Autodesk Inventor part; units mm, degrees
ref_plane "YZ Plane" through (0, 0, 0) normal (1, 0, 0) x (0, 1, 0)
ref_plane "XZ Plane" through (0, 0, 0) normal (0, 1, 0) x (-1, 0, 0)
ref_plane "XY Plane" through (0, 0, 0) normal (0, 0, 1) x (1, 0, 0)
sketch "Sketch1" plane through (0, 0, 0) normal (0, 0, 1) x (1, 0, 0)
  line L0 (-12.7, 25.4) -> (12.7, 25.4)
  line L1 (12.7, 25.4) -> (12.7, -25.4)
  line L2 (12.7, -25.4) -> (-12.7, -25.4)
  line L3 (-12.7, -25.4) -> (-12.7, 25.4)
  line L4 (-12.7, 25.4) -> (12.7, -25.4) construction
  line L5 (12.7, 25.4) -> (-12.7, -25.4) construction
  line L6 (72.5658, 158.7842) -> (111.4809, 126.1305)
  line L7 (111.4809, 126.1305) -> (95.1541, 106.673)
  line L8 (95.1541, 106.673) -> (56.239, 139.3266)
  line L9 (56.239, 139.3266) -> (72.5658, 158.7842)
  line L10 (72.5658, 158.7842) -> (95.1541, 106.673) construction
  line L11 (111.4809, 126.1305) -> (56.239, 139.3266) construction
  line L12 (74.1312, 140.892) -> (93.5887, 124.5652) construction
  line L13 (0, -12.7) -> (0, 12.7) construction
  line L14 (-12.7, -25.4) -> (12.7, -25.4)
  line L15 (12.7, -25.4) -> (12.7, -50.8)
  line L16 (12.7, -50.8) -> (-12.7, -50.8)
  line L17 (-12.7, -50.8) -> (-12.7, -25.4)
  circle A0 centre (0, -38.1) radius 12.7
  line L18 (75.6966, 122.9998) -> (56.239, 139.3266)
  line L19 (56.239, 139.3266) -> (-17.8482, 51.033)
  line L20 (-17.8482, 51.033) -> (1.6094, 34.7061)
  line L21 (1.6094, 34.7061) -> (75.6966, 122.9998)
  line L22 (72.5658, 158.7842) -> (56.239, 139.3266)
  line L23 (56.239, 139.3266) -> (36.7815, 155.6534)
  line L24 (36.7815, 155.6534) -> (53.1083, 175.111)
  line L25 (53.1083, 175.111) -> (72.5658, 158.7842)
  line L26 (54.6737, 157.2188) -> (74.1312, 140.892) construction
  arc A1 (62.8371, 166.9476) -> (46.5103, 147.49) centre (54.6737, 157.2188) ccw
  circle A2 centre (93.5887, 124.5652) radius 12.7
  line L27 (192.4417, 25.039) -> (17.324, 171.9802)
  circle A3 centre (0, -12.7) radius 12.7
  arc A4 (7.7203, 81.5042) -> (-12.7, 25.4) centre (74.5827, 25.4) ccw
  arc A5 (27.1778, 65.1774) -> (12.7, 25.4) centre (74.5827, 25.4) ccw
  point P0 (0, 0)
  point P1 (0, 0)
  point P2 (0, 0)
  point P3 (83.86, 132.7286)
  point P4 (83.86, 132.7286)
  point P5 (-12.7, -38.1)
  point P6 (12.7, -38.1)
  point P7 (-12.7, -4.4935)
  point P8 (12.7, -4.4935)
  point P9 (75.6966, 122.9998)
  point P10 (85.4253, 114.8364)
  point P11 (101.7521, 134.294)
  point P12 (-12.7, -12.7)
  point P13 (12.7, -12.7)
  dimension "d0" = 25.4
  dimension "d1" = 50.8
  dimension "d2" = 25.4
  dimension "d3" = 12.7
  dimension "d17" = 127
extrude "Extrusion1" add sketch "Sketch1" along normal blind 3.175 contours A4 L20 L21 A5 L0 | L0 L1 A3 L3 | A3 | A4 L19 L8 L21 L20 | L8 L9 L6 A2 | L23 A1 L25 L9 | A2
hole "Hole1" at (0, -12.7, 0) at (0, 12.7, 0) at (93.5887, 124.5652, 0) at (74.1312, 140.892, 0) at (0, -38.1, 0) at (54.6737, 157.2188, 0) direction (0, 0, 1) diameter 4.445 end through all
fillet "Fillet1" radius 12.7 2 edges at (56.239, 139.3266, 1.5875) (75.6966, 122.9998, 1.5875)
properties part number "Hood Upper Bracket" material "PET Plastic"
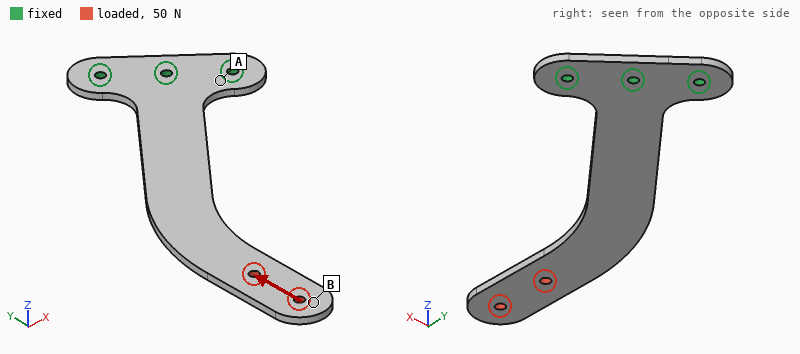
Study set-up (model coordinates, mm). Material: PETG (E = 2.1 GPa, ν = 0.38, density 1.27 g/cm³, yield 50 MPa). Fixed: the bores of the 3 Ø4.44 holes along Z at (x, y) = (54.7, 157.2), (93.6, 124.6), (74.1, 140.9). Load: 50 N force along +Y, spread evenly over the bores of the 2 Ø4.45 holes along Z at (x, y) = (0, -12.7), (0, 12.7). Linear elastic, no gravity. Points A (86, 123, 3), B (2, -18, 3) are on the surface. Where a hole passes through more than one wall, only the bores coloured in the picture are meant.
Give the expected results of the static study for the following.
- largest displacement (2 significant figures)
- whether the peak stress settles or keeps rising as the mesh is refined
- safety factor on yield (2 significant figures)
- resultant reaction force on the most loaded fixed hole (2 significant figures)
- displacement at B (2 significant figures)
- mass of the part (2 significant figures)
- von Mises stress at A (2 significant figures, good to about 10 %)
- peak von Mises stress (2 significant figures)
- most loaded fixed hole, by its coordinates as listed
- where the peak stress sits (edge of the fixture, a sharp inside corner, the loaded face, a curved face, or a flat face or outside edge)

2.7 mm
settles
4.2
88 N
2.6 mm
25 g
2.3 MPa
12 MPa
(54.7, 157.2)
a curved face
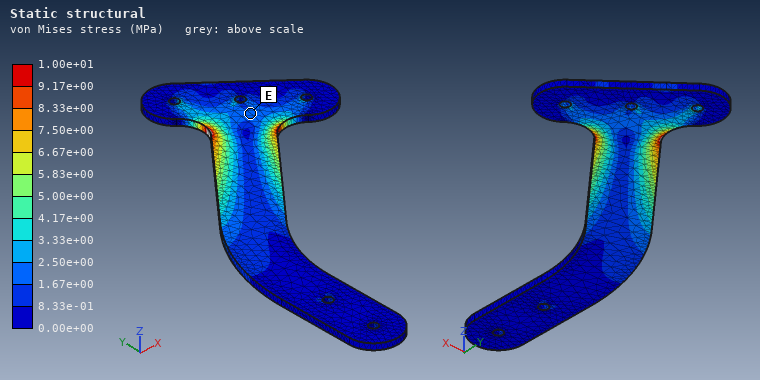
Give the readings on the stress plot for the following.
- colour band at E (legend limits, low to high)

1.67e+00 to 2.50e+00 MPa
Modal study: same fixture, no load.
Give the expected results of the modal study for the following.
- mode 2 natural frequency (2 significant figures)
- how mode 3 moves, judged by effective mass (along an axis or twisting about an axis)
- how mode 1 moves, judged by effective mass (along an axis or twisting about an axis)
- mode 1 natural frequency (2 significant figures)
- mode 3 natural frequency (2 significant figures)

110 Hz
along X
along Z
21 Hz
170 Hz
